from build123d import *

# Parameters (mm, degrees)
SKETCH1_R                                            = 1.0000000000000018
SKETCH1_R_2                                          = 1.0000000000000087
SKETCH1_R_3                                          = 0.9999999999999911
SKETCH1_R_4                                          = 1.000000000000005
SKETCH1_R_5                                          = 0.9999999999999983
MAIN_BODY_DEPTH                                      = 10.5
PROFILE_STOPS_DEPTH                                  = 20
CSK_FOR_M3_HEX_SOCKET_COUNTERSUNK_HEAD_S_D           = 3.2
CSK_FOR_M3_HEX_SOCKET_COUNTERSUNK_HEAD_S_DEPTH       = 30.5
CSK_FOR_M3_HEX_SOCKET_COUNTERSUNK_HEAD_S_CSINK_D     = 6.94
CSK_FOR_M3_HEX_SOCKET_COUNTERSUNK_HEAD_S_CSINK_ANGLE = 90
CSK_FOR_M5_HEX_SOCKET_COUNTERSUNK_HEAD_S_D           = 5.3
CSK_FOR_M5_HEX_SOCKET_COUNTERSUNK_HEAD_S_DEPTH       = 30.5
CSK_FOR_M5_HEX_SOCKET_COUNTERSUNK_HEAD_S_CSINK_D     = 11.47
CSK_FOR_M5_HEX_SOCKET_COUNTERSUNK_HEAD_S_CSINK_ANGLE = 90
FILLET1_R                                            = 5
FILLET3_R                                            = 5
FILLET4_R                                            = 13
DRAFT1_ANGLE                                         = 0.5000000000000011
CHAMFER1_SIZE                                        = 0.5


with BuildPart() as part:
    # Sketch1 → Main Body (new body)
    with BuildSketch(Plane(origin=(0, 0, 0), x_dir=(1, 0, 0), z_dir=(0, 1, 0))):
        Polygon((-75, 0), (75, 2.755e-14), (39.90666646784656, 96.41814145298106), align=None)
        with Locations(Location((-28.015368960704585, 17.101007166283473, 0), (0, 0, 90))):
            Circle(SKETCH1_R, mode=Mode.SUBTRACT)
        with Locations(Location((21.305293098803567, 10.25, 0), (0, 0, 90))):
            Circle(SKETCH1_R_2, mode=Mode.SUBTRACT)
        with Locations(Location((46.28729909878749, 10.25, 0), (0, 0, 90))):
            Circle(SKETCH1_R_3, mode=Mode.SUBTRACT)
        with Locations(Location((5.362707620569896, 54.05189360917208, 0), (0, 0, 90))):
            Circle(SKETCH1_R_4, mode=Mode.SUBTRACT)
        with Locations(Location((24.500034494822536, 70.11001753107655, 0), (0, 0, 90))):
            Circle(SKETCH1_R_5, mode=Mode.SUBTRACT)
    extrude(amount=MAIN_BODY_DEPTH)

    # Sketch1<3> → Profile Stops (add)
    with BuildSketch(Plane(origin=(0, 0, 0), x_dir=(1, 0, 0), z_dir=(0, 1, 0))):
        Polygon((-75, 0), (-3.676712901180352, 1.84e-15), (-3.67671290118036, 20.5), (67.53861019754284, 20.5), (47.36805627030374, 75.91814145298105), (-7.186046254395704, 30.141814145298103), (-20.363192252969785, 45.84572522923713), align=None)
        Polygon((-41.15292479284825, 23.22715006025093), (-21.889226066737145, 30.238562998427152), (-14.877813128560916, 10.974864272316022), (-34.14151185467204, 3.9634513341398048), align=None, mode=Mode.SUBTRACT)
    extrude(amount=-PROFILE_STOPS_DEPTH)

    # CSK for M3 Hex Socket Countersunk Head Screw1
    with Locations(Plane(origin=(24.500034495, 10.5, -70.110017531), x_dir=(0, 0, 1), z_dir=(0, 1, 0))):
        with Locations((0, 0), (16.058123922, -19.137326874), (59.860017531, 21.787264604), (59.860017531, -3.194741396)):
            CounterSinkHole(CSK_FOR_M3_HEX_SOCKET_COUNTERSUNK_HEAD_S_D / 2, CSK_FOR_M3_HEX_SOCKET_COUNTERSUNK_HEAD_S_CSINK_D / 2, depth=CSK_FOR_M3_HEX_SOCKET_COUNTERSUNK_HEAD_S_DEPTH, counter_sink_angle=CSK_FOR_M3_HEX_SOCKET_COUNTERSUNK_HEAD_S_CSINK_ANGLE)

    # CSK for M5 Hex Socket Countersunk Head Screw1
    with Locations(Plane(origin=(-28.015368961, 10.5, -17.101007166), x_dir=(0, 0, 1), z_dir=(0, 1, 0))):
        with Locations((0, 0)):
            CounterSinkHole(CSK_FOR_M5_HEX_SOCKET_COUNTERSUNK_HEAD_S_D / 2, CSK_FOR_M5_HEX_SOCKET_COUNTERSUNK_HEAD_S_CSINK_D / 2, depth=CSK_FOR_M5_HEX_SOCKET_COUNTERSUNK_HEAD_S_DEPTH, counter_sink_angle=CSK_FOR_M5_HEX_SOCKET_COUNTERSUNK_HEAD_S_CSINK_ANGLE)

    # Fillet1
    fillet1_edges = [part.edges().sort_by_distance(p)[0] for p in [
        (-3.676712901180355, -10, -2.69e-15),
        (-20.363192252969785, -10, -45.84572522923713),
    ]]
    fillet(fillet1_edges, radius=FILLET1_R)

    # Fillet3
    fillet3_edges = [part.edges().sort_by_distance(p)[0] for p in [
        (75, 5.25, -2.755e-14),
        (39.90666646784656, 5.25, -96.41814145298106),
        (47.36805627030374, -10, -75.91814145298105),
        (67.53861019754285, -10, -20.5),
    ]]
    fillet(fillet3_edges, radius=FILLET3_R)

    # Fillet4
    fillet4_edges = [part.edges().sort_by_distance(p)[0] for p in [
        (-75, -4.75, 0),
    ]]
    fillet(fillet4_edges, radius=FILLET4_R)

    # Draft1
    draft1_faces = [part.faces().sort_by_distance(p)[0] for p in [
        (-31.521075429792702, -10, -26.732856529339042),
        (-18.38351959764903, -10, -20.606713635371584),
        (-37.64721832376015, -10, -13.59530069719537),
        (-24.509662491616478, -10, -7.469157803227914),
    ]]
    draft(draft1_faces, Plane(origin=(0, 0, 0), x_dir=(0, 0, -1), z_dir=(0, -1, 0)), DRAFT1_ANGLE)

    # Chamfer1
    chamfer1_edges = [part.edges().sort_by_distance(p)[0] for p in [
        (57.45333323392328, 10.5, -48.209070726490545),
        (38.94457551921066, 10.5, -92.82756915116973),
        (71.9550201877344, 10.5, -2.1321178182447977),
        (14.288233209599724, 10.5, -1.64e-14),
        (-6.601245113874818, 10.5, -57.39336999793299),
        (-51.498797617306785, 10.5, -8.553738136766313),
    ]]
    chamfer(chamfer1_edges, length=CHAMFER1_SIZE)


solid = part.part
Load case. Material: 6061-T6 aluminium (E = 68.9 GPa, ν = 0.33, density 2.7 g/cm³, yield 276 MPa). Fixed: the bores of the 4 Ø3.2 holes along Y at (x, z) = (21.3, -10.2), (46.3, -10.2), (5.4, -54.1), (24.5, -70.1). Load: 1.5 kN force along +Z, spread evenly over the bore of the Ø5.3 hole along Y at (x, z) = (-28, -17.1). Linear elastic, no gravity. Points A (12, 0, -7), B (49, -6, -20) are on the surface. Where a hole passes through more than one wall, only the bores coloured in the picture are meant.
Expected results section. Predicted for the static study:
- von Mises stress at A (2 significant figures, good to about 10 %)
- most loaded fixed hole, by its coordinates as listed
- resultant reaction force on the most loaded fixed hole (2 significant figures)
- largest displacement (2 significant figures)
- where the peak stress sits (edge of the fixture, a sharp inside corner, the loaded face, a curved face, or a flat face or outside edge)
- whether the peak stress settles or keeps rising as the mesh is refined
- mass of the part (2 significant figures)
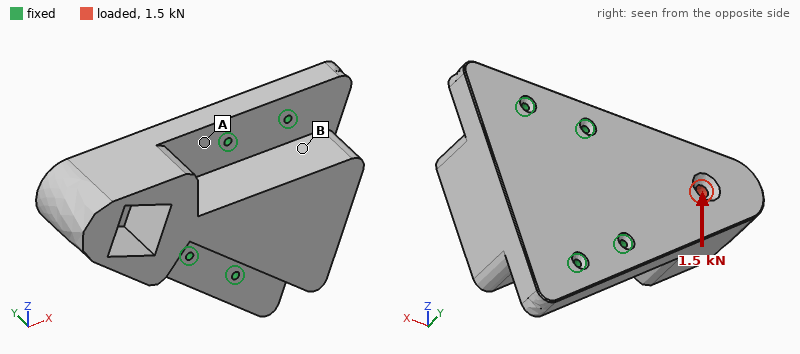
6.5 MPa
(5.4, -54.1)
1.3 kN
11 µm
edge of the fixture
keeps rising
380 g
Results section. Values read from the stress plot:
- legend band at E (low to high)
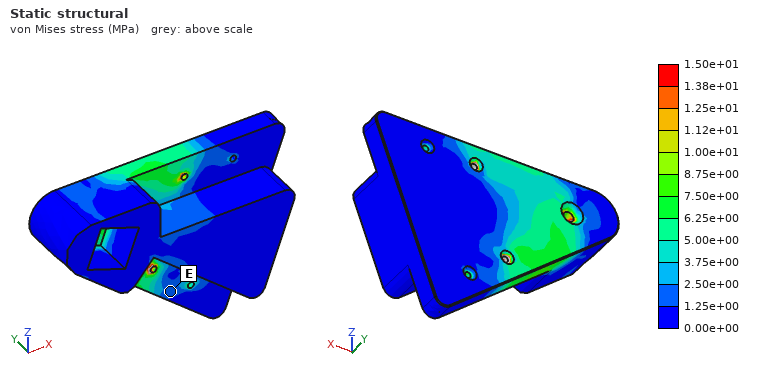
1.25e+00 to 2.50e+00 MPa
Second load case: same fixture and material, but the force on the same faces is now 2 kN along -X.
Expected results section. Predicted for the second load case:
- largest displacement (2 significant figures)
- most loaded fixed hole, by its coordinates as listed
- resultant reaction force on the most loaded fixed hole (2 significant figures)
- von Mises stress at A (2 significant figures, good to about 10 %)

6.6 µm
(21.3, -10.2)
1.2 kN
7.5 MPa
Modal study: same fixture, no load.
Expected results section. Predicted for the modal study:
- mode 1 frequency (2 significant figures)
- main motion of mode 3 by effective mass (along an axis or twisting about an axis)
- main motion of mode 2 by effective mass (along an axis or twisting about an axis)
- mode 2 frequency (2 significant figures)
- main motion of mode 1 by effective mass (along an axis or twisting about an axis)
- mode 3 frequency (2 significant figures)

2600 Hz
along Y
along Z
6000 Hz
along Y
6700 Hz
